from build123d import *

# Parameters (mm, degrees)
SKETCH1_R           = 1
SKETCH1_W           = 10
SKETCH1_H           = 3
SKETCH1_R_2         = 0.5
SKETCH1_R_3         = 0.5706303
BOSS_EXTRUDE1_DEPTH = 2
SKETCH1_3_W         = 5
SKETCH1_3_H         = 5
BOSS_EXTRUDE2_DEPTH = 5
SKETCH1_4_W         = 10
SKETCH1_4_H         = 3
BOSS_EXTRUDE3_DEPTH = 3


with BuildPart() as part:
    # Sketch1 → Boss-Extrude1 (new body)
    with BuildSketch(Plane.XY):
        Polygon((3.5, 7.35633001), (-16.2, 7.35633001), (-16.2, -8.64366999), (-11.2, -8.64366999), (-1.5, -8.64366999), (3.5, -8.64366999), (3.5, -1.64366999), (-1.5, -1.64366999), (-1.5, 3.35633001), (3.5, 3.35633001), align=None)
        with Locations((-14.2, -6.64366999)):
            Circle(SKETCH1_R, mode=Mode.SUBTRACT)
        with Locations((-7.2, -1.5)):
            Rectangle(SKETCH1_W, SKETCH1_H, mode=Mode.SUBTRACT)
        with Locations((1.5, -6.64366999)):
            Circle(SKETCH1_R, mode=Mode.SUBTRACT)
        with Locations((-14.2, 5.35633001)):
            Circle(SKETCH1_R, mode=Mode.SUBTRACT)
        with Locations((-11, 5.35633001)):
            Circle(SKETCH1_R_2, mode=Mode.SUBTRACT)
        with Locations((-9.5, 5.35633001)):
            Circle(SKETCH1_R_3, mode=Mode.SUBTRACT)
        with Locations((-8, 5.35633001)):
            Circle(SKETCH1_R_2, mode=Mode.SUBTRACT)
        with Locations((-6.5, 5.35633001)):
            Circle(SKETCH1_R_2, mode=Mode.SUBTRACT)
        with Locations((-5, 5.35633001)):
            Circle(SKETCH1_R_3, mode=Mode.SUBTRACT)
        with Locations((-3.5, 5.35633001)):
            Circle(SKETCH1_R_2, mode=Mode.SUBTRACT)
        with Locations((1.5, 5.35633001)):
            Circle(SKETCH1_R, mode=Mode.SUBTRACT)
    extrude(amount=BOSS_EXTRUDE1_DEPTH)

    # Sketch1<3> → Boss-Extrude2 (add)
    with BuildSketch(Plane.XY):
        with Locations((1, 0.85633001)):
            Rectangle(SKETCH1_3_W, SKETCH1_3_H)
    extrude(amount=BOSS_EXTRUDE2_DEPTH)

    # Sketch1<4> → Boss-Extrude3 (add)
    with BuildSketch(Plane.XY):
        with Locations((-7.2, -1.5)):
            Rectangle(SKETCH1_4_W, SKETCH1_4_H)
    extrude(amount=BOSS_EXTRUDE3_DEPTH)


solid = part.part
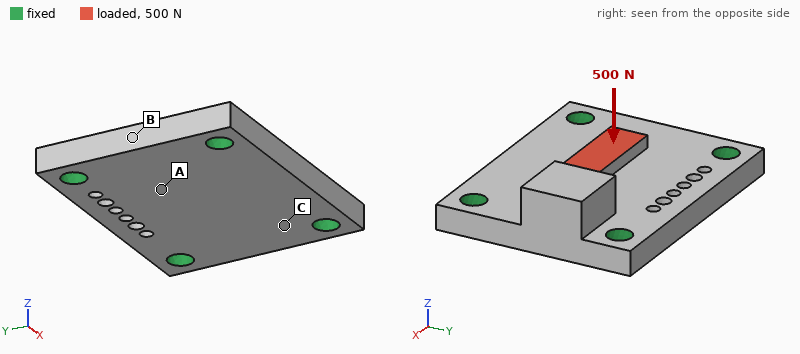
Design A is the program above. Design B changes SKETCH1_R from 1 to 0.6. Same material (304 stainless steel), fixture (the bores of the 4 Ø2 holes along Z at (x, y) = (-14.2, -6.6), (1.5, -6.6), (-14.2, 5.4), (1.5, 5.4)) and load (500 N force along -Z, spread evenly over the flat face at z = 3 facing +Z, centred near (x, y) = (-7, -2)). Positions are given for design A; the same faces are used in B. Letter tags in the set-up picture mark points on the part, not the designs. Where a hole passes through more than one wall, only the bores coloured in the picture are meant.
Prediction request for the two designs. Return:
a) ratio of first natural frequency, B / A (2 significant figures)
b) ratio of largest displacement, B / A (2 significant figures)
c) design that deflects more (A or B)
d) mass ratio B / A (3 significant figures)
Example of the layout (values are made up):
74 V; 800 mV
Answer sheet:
0.87; 1.2; B; 1.02
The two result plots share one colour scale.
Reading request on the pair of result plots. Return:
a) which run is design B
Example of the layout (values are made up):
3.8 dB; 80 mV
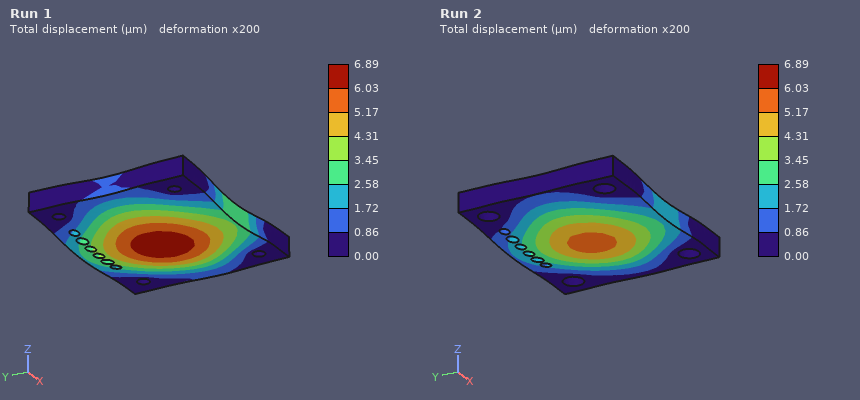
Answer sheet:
Run 1
